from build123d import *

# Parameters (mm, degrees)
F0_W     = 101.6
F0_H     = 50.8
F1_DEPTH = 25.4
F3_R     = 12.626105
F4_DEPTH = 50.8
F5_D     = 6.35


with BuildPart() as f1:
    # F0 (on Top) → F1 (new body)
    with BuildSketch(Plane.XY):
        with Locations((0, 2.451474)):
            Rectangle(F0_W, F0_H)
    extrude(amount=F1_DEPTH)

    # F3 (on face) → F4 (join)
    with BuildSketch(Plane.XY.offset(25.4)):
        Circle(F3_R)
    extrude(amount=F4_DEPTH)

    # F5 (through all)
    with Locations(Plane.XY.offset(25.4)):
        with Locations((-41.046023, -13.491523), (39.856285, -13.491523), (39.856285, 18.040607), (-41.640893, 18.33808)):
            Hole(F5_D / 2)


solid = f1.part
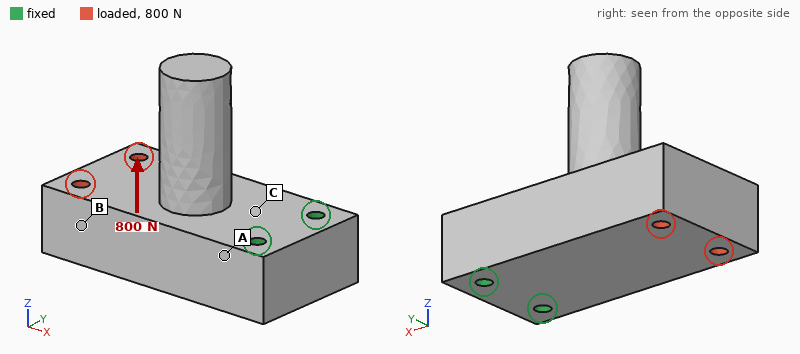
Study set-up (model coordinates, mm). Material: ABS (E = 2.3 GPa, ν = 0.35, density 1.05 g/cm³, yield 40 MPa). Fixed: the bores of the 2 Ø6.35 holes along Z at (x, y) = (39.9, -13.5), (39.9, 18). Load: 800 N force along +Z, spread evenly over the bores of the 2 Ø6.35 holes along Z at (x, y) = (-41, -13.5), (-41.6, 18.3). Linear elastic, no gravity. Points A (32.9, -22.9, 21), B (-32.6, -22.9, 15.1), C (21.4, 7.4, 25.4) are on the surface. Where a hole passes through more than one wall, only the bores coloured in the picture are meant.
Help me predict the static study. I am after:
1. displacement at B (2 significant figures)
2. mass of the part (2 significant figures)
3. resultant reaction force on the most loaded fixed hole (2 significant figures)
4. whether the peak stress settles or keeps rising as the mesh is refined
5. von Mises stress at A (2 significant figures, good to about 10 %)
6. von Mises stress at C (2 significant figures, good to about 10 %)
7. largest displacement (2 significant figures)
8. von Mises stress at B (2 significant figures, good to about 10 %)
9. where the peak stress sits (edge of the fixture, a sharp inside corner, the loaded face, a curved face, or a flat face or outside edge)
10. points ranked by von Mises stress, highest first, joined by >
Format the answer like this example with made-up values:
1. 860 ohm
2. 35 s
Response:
1. 0.85 mm
2. 160 g
3. 400 N
4. keeps rising
5. 4.7 MPa
6. 8.4 MPa
7. 1.2 mm
8. 2.1 MPa
9. edge of the fixture
10. C > A > B
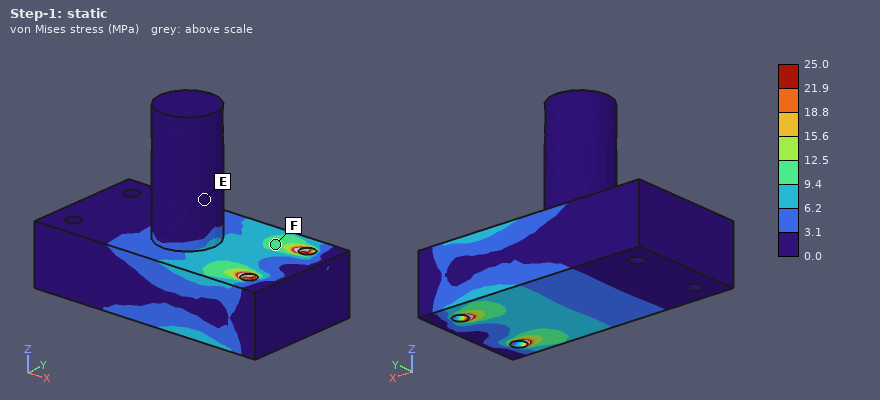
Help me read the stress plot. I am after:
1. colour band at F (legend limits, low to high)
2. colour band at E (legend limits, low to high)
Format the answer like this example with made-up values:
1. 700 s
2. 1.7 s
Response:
1. 9.4 to 12.5 MPa
2. 0.0 to 3.1 MPa
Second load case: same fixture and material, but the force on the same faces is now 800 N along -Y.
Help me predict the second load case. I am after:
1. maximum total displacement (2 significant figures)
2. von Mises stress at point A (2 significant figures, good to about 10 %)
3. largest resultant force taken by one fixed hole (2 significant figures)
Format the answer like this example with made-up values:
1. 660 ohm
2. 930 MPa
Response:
1. 0.37 mm
2. 3.7 MPa
3. 1.9 kN
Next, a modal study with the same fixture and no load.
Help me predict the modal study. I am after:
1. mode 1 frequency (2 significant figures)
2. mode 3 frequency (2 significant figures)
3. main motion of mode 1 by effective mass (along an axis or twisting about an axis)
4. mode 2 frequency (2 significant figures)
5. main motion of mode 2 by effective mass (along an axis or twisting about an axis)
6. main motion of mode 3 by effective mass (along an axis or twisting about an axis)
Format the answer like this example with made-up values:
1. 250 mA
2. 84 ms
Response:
1. 600 Hz
2. 1300 Hz
3. along Z
4. 1000 Hz
5. along Y
6. along Y
